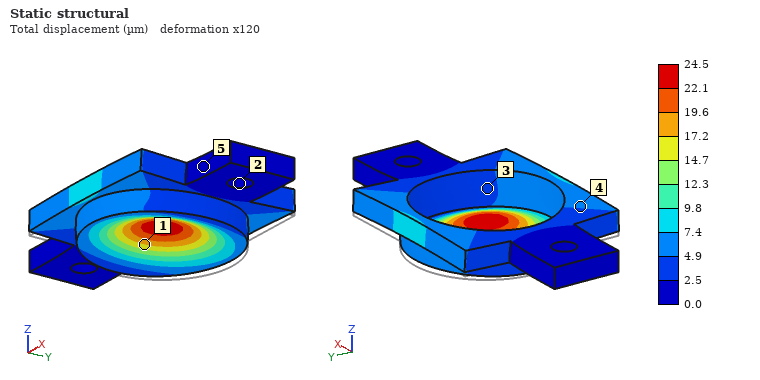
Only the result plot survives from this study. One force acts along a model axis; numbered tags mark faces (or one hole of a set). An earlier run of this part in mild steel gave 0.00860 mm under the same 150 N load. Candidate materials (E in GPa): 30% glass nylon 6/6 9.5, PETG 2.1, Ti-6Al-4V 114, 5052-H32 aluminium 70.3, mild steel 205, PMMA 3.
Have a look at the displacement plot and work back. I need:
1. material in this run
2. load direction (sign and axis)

5052-H32 aluminium
+Z
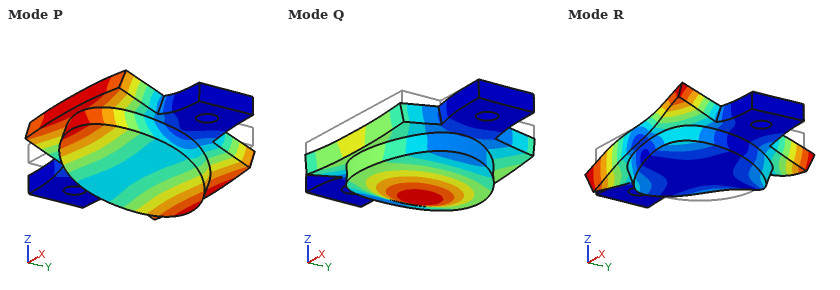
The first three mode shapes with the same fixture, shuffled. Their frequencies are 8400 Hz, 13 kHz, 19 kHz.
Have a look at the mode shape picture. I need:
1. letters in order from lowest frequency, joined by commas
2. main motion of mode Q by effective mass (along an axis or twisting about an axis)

P, Q, R
along Z
